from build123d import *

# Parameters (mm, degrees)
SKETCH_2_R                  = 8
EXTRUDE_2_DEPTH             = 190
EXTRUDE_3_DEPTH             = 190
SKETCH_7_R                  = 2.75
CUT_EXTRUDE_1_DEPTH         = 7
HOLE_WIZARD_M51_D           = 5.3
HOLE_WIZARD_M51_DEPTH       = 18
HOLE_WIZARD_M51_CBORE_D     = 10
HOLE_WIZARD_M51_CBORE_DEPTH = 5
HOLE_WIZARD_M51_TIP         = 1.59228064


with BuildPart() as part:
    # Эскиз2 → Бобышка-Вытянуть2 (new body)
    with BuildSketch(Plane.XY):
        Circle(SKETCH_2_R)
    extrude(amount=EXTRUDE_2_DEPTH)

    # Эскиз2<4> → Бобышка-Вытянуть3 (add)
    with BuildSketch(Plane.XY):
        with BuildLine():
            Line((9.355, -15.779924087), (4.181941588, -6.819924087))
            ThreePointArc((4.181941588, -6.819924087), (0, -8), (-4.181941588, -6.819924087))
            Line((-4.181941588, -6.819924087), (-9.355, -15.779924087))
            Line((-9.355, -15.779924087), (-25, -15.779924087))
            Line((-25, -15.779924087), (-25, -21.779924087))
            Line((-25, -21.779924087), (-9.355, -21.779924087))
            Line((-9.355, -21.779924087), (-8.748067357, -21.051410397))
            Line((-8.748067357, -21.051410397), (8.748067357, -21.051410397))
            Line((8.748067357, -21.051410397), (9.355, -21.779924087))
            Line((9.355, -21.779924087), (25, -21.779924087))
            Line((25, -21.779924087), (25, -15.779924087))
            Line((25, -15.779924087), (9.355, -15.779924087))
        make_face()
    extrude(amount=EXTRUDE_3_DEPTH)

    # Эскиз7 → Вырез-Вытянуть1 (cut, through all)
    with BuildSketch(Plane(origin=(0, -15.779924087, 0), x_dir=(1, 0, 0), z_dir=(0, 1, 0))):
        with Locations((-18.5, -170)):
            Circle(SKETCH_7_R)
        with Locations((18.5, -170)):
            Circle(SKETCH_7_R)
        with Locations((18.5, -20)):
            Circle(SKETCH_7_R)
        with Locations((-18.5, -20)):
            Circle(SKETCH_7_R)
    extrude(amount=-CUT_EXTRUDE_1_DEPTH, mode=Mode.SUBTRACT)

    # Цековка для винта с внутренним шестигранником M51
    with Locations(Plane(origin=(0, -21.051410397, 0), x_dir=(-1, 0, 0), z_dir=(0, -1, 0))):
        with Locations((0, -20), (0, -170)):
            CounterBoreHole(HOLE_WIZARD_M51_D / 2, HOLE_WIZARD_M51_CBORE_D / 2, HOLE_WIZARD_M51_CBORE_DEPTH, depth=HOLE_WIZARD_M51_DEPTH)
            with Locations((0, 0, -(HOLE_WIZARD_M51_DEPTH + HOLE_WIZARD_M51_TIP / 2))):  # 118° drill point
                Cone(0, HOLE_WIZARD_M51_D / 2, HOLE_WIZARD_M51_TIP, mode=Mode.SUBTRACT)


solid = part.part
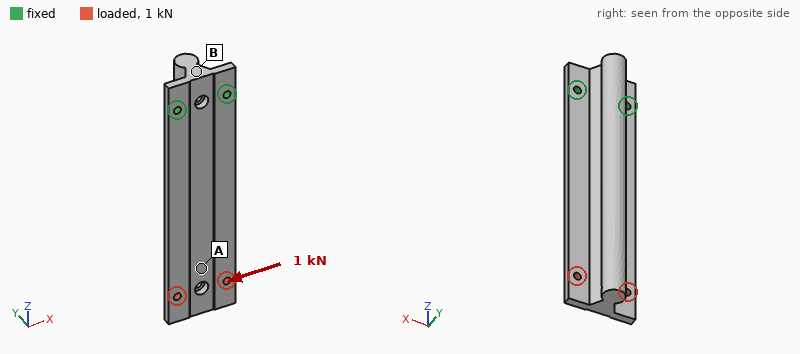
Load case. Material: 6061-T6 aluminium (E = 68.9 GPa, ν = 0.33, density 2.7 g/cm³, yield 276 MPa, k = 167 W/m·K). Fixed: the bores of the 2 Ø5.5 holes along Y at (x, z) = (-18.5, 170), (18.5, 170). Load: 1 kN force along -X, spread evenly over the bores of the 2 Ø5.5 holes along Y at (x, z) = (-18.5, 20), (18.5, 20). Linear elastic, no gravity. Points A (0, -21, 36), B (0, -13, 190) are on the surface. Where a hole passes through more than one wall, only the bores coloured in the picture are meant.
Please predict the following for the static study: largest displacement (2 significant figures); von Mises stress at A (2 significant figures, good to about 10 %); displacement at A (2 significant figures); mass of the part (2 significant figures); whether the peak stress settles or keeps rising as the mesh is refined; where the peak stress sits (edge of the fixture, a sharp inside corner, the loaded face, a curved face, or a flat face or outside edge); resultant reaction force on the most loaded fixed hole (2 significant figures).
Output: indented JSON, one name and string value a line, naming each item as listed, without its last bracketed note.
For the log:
{
  "largest displacement": "0.33 mm",
  "von Mises stress at A": "10 MPa",
  "displacement at A": "0.23 mm",
  "mass of the part": "300 g",
  "whether the peak stress settles or keeps rising as the mesh is refined": "keeps rising",
  "where the peak stress sits": "edge of the fixture",
  "resultant reaction force on the most loaded fixed hole": "3.9 kN"
}
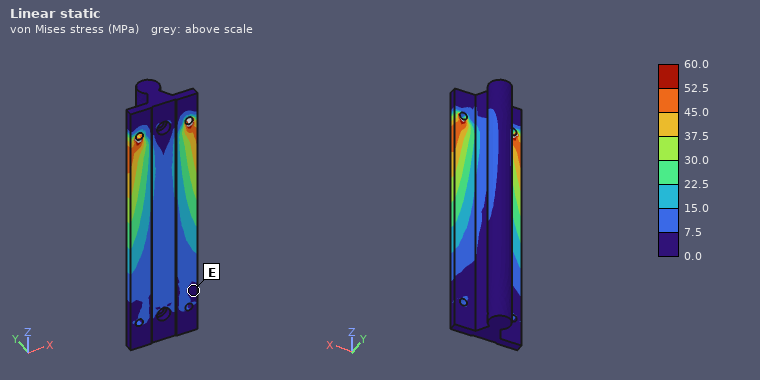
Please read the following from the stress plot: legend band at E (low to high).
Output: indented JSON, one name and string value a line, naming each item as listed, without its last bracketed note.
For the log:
{
  "legend band at E": "0.0 to 7.5 MPa"
}
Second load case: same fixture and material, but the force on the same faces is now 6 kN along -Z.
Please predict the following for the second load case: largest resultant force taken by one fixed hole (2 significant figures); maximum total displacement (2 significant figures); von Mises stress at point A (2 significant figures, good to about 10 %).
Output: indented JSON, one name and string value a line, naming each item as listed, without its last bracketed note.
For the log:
{
  "largest resultant force taken by one fixed hole": "3.0 kN",
  "maximum total displacement": "0.18 mm",
  "von Mises stress at point A": "13 MPa"
}
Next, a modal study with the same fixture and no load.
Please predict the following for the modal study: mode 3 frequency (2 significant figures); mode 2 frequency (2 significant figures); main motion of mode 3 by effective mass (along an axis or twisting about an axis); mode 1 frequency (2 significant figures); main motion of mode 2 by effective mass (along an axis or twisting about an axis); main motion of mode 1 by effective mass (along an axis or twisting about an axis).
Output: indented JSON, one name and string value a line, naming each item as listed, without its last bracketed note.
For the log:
{
  "mode 3 frequency": "1900 Hz",
  "mode 2 frequency": "970 Hz",
  "main motion of mode 3 by effective mass": "twisting about Z",
  "mode 1 frequency": "310 Hz",
  "main motion of mode 2 by effective mass": "along X",
  "main motion of mode 1 by effective mass": "along Y"
}
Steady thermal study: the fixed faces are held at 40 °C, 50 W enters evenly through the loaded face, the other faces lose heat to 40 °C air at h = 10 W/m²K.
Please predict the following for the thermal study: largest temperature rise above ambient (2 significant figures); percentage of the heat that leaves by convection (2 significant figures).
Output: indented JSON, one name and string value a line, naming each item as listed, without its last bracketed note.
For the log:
{
  "largest temperature rise above ambient": "79 K",
  "percentage of the heat that leaves by convection": "23 %"
}
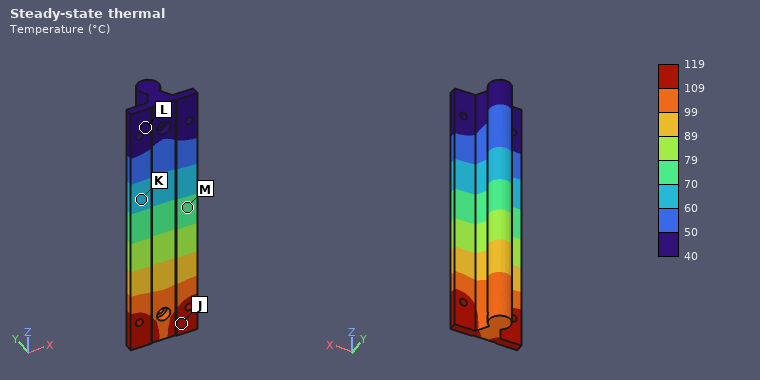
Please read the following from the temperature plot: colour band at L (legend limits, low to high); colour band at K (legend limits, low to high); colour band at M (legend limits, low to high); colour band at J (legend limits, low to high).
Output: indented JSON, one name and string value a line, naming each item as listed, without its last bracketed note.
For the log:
{
  "colour band at L": "40 to 50 °C",
  "colour band at K": "60 to 70 °C",
  "colour band at M": "70 to 79 °C",
  "colour band at J": "109 to 119 °C"
}
